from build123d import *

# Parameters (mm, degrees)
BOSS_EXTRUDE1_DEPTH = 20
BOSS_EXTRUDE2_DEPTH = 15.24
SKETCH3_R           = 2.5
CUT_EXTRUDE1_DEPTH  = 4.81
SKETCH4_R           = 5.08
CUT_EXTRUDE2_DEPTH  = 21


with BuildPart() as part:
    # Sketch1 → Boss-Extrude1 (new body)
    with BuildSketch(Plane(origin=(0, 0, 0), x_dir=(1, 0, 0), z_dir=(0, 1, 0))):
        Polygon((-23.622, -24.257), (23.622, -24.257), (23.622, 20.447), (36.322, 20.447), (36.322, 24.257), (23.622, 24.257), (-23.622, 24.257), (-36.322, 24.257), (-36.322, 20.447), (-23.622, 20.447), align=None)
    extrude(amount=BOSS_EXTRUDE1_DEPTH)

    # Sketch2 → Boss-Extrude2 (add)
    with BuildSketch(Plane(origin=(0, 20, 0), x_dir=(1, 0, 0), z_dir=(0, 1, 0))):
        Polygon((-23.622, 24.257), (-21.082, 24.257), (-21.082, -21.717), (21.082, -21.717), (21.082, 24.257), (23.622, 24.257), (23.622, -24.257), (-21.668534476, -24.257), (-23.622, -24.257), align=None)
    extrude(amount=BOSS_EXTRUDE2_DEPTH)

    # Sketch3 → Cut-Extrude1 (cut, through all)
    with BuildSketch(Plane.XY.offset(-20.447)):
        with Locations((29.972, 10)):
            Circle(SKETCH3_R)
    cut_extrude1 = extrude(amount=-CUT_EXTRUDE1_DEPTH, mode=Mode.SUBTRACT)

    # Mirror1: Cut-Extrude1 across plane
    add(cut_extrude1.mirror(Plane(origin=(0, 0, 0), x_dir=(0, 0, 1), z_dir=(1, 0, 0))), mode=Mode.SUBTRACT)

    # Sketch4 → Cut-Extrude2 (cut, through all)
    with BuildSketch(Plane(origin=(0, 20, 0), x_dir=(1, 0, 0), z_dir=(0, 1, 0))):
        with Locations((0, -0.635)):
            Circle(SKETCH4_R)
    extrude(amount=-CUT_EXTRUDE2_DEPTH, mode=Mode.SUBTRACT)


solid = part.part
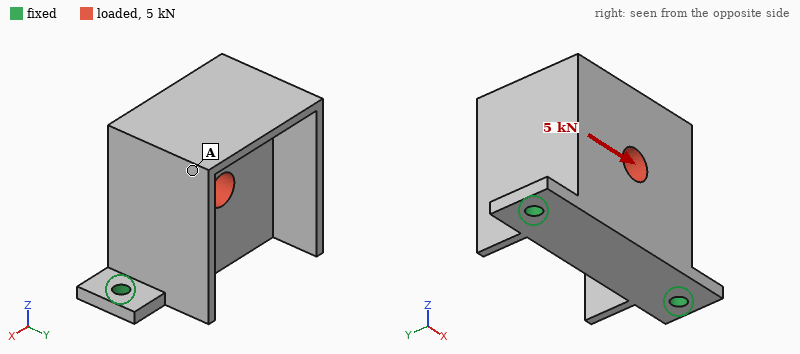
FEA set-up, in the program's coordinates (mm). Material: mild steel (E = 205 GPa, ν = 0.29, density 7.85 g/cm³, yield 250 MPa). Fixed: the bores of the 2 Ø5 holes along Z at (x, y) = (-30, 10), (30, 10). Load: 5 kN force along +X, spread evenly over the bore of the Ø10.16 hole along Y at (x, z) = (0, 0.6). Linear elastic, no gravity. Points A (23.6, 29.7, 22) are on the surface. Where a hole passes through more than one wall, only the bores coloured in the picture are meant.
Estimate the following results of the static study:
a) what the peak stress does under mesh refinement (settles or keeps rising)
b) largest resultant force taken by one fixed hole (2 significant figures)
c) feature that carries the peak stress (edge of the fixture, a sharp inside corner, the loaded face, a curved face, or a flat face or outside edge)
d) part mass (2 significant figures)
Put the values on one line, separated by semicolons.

keeps rising; 3.3 kN; edge of the fixture; 400 g
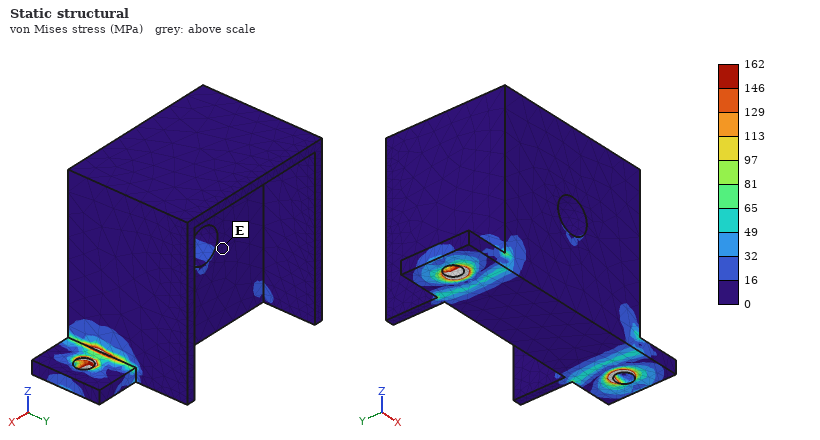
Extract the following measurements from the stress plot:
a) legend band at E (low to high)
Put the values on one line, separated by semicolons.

0 to 16 MPa
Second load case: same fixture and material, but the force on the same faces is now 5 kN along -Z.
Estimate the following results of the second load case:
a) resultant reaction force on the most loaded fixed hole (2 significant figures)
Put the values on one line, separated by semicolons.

2.8 kN
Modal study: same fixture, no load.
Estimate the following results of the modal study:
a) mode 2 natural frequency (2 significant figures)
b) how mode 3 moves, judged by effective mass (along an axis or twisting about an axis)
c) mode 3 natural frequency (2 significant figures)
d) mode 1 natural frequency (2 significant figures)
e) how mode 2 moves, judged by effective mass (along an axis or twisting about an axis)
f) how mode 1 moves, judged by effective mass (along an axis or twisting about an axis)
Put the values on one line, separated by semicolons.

4400 Hz; along Z; 5400 Hz; 930 Hz; along X; along Y
